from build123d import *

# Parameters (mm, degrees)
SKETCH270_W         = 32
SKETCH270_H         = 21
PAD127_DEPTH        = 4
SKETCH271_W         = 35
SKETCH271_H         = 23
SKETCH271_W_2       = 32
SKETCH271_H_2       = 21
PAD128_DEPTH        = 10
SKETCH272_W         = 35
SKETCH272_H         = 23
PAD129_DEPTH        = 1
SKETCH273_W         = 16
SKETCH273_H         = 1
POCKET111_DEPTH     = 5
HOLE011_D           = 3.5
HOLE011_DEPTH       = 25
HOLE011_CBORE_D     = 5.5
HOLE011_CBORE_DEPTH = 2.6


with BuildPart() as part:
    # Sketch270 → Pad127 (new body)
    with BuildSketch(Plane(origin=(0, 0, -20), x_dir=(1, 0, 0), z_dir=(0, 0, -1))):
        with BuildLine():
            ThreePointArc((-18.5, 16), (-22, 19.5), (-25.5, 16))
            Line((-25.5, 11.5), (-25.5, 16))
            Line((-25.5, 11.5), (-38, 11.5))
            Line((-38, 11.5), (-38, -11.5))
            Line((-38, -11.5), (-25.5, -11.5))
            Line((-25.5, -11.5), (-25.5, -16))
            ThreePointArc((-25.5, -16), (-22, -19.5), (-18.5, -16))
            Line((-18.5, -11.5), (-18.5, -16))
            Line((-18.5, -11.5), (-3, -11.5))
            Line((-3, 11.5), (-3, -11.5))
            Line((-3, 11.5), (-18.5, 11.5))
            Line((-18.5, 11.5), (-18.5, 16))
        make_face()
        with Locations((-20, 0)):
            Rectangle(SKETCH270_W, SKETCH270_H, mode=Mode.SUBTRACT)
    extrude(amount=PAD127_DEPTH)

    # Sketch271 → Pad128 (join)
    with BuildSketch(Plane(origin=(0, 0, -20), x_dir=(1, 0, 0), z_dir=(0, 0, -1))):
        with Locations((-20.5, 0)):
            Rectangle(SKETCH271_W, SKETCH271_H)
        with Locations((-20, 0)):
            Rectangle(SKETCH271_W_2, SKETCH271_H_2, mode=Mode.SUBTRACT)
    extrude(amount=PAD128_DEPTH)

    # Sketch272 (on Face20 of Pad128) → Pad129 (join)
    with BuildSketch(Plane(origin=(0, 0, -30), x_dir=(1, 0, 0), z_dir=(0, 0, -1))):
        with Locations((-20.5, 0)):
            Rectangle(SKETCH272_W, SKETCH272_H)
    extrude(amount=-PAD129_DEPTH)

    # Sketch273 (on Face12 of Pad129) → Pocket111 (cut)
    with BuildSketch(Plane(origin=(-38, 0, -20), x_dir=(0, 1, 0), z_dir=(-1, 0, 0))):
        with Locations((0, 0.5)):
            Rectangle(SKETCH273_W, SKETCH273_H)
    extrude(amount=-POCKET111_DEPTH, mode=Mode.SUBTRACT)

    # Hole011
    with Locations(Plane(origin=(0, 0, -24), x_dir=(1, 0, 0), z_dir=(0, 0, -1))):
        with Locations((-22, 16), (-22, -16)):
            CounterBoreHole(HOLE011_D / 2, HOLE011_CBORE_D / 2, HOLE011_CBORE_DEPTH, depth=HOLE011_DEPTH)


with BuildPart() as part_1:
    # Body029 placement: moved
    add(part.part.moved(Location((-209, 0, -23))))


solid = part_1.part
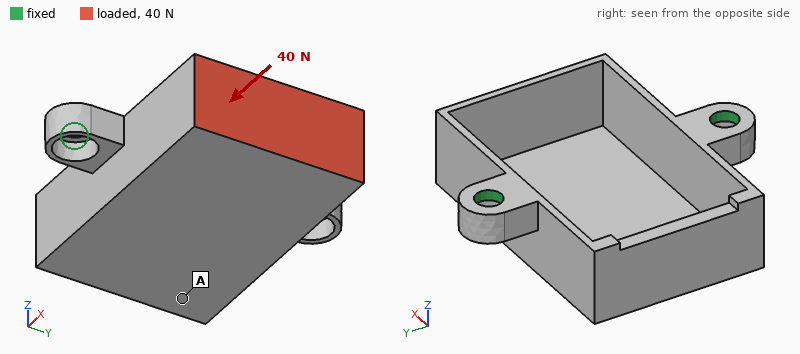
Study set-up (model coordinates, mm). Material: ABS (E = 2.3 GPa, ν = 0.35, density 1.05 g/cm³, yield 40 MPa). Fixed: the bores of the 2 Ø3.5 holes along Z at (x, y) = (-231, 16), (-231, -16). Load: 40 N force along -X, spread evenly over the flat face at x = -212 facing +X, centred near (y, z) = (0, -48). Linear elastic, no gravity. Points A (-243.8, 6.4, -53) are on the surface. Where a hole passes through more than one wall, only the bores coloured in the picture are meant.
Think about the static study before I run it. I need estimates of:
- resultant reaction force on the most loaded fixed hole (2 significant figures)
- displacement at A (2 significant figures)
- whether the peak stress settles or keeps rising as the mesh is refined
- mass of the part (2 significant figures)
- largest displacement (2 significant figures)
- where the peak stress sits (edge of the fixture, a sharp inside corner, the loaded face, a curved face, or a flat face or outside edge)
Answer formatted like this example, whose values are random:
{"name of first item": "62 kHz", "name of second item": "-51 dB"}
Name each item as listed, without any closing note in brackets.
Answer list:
{"resultant reaction force on the most loaded fixed hole": "20 N", "displacement at A": "0.17 mm", "whether the peak stress settles or keeps rising as the mesh is refined": "keeps rising", "mass of the part": "2.3 g", "largest displacement": "0.54 mm", "where the peak stress sits": "edge of the fixture"}
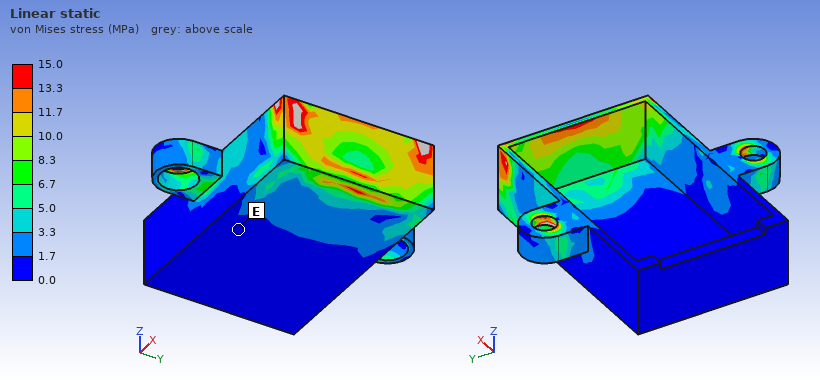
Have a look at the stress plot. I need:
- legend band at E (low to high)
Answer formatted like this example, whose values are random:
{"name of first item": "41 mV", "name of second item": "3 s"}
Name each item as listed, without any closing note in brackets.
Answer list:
{"legend band at E": "0.0 to 1.7 MPa"}
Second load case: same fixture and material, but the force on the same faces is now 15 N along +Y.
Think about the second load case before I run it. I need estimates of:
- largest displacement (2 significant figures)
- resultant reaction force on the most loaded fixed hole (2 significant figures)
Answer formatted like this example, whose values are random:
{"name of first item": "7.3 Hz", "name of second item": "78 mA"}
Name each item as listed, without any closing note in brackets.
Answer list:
{"largest displacement": "0.55 mm", "resultant reaction force on the most loaded fixed hole": "13 N"}
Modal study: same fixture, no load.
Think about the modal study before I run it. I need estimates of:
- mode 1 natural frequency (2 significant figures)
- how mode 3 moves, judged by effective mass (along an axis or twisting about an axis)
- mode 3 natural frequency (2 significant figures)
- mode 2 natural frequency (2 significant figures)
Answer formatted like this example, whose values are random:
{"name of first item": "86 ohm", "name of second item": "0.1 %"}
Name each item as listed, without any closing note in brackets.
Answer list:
{"mode 1 natural frequency": "960 Hz", "how mode 3 moves, judged by effective mass": "along Y", "mode 3 natural frequency": "1500 Hz", "mode 2 natural frequency": "1200 Hz"}
